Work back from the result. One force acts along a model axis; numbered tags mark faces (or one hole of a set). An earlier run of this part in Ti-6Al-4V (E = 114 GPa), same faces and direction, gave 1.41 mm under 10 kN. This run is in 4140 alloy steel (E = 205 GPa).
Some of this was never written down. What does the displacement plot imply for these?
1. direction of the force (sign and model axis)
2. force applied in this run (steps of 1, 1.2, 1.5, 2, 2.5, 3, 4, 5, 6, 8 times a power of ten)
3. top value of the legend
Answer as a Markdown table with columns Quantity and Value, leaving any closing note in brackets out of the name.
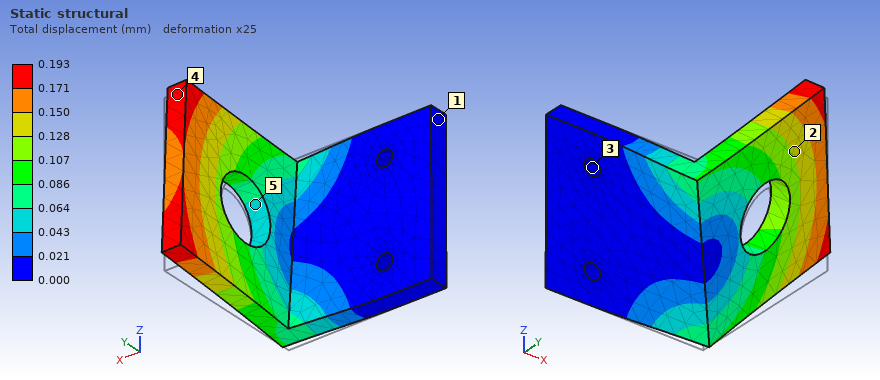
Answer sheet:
| Quantity | Value |
|---|---|
| direction of the force | +Z |
| force applied in this run | 2.5 kN |
| top value of the legend | 0.193 mm |
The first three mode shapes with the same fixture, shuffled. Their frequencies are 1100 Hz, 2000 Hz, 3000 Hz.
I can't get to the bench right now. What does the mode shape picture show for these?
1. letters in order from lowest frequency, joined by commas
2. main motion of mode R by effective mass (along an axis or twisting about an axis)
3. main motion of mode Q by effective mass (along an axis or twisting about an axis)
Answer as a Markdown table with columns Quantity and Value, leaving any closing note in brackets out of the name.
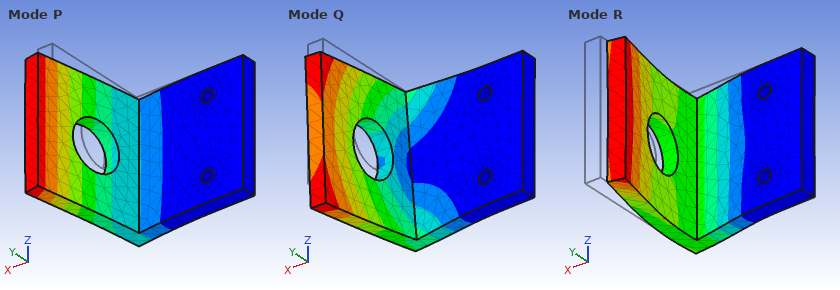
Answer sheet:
| Quantity | Value |
|---|---|
| letters in order from lowest frequency, joined by commas | P, Q, R |
| main motion of mode R by effective mass | along Y |
| main motion of mode Q by effective mass | along Z |
